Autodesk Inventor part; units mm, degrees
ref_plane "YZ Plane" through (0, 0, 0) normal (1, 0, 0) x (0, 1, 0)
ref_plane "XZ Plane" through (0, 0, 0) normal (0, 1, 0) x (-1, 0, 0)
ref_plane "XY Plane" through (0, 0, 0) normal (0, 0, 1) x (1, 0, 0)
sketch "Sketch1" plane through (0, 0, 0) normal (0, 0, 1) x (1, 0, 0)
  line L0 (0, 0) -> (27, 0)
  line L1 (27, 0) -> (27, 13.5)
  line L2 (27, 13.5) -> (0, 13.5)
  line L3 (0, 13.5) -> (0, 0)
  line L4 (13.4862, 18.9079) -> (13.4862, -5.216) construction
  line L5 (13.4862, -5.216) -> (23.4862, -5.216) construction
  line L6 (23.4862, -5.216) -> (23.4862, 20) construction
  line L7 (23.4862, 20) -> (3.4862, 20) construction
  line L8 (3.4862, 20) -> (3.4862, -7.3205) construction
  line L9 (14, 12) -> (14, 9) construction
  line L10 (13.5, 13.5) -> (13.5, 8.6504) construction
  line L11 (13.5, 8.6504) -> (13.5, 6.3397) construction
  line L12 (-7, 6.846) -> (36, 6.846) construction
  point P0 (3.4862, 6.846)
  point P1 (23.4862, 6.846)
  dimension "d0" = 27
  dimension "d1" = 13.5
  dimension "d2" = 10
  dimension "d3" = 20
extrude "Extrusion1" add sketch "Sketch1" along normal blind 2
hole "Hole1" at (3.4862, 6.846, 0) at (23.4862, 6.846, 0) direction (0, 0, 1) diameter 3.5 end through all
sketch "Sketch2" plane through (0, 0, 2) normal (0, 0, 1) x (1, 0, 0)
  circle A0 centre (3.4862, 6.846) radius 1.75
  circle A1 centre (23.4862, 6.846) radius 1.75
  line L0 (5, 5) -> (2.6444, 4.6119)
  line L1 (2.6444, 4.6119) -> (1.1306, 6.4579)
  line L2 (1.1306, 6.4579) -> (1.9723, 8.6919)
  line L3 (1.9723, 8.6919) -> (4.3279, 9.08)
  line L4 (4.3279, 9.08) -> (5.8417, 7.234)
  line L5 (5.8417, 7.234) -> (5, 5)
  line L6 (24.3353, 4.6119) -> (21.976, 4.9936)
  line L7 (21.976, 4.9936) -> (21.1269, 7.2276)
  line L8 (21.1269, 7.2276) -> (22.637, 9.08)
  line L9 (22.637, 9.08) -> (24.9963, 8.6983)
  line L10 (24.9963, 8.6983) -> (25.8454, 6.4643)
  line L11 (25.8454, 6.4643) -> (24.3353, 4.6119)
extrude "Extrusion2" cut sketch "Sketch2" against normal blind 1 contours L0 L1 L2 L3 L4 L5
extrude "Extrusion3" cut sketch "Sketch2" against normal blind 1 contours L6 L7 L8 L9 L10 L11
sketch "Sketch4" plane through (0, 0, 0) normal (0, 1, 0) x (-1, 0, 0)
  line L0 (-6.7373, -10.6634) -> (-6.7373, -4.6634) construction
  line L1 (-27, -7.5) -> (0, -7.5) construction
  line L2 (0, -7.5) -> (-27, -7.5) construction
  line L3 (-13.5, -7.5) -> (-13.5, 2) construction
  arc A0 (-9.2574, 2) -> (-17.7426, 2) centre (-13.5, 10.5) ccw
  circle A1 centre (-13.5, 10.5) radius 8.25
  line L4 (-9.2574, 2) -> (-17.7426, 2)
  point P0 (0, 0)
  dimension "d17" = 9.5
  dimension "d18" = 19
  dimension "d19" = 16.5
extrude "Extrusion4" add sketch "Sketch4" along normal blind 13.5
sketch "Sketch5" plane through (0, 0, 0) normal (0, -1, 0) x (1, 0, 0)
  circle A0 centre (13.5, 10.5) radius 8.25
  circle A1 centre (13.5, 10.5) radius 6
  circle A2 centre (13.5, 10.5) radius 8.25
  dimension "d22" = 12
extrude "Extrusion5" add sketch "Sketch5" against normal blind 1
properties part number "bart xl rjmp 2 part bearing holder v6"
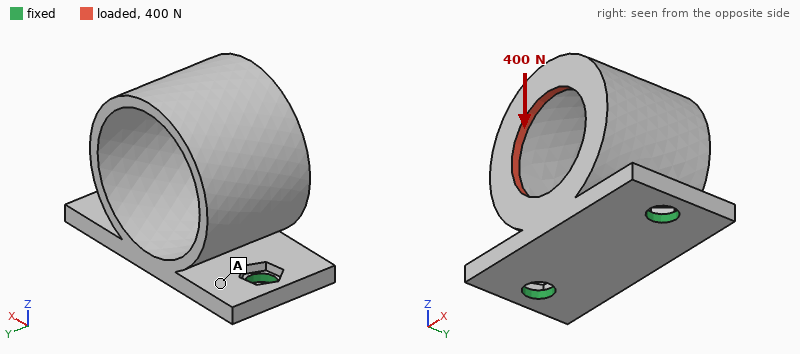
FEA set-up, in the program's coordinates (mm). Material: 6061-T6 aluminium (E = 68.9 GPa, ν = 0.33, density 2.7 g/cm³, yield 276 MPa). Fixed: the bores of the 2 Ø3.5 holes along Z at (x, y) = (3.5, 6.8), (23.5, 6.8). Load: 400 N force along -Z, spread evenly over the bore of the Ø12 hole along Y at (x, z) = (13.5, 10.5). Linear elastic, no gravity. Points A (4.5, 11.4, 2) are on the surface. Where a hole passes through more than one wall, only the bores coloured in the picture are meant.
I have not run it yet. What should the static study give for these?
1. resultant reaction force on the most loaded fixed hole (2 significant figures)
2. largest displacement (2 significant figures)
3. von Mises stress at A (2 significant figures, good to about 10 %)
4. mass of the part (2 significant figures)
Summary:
270 N
0.22 mm
42 MPa
4.4 g
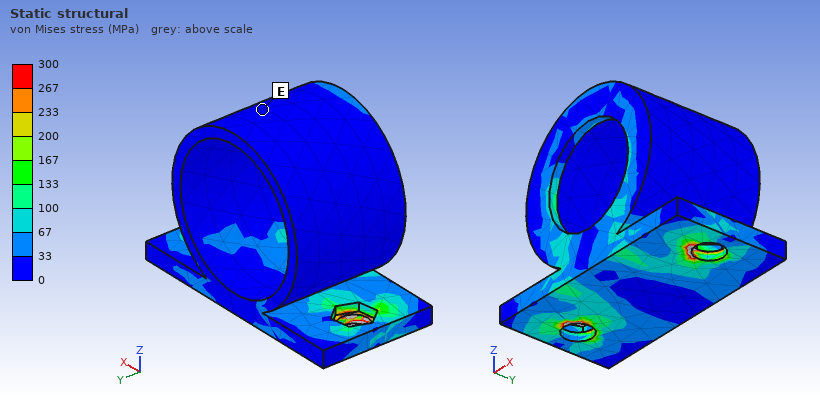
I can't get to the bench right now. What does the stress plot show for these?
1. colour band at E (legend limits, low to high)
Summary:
0 to 33 MPa
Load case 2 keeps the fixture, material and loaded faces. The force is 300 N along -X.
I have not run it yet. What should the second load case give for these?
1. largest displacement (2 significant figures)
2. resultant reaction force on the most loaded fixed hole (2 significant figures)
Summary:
0.17 mm
260 N
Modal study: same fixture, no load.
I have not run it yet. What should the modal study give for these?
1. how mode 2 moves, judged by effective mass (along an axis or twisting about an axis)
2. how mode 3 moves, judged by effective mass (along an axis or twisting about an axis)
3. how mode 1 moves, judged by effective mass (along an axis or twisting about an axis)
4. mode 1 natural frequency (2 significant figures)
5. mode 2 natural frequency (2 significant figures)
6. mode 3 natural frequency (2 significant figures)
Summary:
along X
along Z
along Y
3700 Hz
4200 Hz
9600 Hz
